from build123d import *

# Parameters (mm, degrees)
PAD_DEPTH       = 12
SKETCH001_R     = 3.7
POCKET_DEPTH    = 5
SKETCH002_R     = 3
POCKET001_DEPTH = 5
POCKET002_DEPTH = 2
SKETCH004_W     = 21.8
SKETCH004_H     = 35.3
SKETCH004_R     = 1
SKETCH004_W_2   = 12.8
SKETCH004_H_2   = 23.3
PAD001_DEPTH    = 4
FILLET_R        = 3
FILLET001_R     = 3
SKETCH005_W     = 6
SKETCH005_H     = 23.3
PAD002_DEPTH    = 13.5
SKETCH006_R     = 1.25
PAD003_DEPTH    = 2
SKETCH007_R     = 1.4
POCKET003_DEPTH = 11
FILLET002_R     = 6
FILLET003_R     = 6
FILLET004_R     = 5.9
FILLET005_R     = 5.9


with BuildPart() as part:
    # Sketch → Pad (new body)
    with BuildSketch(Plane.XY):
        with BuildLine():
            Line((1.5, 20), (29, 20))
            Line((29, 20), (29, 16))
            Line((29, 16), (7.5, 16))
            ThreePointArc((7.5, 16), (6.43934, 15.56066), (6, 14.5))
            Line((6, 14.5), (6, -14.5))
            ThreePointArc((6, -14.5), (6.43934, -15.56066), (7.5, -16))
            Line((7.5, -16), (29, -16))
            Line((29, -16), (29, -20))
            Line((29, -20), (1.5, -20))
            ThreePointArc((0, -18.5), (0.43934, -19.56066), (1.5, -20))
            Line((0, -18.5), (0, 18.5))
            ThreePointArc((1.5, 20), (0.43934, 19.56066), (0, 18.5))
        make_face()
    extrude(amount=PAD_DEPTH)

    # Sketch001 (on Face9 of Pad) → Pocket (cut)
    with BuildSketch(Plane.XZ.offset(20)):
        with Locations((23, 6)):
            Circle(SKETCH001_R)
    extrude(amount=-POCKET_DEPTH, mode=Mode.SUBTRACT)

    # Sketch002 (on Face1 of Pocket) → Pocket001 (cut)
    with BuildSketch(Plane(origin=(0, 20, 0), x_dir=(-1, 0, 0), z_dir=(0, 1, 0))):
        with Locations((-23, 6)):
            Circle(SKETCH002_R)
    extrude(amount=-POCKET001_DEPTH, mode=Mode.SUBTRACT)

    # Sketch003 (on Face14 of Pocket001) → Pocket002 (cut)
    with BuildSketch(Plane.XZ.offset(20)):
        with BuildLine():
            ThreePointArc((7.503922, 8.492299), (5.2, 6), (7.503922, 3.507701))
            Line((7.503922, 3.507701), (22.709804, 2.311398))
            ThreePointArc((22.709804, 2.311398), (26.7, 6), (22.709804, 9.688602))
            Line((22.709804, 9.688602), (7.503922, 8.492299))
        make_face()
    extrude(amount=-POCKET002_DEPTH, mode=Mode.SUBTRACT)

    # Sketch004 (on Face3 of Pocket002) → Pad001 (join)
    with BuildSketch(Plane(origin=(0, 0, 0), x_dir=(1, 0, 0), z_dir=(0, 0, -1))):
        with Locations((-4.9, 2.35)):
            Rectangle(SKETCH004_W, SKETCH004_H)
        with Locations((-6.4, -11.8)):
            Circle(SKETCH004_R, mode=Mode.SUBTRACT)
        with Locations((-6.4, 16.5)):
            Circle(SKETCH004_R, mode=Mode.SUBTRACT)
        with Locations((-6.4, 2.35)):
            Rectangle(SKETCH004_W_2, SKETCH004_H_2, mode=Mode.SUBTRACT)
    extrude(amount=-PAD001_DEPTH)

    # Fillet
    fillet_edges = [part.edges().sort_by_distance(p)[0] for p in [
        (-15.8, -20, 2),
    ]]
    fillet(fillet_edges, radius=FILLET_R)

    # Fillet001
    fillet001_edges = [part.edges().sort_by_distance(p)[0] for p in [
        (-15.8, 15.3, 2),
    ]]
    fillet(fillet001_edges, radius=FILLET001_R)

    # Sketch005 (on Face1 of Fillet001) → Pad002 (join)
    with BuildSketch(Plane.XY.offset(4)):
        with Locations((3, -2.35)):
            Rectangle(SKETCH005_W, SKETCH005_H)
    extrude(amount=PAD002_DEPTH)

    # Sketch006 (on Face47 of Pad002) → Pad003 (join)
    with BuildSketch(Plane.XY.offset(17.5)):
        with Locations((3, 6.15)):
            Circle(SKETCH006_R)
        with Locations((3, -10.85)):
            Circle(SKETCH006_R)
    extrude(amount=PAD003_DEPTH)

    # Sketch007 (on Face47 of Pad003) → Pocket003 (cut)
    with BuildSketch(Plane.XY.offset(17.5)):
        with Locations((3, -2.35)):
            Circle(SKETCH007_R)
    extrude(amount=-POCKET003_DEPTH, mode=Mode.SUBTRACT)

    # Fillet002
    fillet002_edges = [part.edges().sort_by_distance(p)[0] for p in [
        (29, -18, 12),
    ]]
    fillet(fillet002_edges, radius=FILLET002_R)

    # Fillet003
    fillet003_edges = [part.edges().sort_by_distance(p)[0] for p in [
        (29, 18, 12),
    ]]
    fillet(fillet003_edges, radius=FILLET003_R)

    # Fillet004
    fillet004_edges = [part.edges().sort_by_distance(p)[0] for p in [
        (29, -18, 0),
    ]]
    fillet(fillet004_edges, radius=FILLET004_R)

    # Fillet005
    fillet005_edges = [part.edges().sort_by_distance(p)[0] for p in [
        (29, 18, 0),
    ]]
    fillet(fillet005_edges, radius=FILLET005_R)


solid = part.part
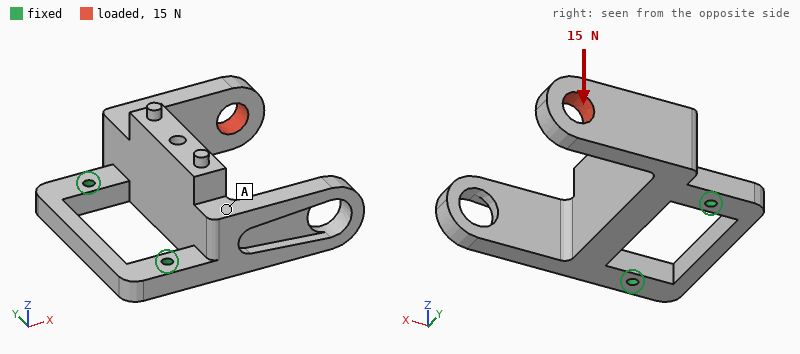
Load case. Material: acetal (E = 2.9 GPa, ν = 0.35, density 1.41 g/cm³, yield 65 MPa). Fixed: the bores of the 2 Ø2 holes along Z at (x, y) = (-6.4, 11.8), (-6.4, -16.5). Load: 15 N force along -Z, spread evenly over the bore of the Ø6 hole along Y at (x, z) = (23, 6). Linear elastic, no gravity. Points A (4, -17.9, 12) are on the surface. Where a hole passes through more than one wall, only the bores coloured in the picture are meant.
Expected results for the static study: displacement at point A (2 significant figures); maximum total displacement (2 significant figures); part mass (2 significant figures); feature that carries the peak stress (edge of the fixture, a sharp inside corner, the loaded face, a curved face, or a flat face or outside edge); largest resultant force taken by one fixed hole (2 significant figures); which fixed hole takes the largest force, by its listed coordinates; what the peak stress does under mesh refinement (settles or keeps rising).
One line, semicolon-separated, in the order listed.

0.15 mm; 0.70 mm; 8.8 g; edge of the fixture; 17 N; (-6.4, 11.8); keeps rising
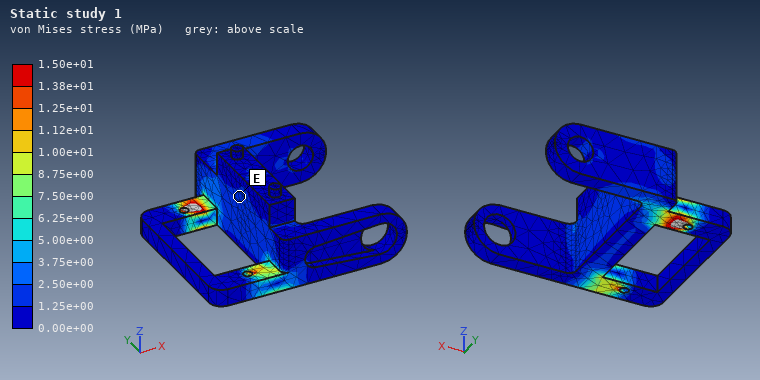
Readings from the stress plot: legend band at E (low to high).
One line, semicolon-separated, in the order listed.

1.25e+00 to 2.50e+00 MPa
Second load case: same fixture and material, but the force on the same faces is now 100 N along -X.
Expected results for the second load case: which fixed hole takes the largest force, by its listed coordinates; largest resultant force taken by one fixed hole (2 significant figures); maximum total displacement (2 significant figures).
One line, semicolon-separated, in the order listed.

(-6.4, 11.8); 120 N; 0.73 mm
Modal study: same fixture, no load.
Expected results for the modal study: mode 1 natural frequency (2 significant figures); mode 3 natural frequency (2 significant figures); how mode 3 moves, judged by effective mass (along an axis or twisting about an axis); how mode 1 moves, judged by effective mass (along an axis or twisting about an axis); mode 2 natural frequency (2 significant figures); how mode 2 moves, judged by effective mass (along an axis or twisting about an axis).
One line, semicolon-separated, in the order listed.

640 Hz; 1500 Hz; along Y; along Z; 1400 Hz; along Y
